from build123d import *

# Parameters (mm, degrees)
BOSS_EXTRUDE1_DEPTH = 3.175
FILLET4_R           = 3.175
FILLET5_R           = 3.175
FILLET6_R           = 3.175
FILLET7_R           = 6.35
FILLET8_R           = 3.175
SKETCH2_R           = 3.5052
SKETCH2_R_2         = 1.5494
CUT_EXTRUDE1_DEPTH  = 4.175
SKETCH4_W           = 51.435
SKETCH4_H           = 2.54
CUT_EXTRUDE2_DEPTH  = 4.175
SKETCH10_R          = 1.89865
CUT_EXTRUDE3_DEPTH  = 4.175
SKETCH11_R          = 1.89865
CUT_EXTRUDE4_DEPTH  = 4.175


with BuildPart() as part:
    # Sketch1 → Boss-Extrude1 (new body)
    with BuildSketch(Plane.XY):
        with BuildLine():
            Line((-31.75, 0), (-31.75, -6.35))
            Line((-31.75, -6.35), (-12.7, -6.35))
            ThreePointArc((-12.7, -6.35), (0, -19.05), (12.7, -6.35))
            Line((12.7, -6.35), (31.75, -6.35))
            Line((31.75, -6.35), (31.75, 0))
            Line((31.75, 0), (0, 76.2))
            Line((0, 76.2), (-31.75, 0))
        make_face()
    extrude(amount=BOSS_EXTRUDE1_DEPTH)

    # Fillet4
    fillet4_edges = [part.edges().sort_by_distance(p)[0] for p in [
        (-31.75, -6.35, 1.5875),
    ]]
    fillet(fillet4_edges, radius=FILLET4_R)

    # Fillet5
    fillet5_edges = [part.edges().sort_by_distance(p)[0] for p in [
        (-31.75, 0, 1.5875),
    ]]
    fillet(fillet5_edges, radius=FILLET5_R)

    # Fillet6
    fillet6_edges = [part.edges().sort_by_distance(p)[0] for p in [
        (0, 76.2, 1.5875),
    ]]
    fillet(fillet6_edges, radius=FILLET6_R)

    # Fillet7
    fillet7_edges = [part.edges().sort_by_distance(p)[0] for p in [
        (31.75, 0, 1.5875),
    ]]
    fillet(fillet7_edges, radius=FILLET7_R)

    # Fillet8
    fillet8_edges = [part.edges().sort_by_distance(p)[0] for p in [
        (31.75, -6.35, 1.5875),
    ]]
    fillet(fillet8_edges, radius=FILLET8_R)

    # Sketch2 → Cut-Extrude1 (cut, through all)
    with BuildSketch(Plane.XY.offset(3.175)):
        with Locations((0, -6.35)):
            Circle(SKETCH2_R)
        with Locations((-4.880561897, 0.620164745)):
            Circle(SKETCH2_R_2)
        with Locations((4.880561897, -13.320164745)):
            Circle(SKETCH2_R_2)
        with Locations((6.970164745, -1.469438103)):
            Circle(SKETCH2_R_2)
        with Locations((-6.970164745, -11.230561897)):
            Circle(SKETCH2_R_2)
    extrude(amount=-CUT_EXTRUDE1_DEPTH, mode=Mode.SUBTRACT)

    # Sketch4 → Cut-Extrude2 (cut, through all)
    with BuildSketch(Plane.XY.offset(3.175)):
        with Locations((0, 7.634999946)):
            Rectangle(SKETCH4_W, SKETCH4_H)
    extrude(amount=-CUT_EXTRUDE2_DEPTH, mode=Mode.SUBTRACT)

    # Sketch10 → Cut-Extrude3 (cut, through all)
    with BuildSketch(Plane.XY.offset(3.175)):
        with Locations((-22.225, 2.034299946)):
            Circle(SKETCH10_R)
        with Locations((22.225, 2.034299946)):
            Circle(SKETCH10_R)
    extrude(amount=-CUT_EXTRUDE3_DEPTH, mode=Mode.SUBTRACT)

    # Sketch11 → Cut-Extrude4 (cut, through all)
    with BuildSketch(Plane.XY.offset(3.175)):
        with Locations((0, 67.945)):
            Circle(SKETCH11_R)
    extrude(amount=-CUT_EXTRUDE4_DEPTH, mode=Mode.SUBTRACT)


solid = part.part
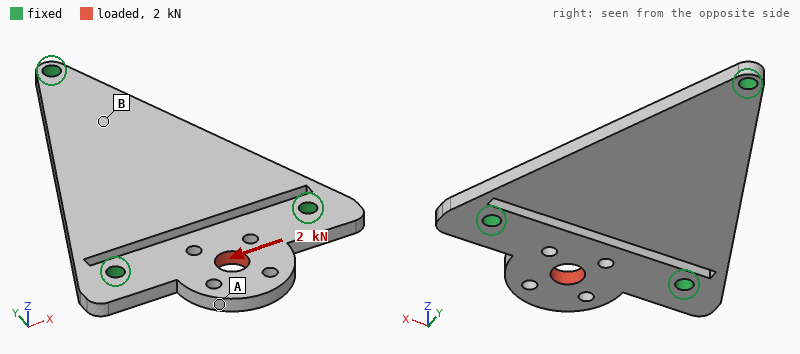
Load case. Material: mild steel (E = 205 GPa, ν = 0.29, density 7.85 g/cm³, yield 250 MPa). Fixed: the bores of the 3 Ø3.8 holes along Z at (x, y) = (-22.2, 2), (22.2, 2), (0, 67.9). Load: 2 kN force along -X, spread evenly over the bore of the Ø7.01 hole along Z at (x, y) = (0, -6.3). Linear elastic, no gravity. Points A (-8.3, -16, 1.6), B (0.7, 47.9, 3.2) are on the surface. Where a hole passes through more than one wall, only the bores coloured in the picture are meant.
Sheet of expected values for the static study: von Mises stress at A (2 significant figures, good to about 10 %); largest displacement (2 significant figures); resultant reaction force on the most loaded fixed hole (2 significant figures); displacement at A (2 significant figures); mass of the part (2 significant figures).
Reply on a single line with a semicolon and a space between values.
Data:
14 MPa; 5.0 µm; 1.1 kN; 4.4 µm; 70 g
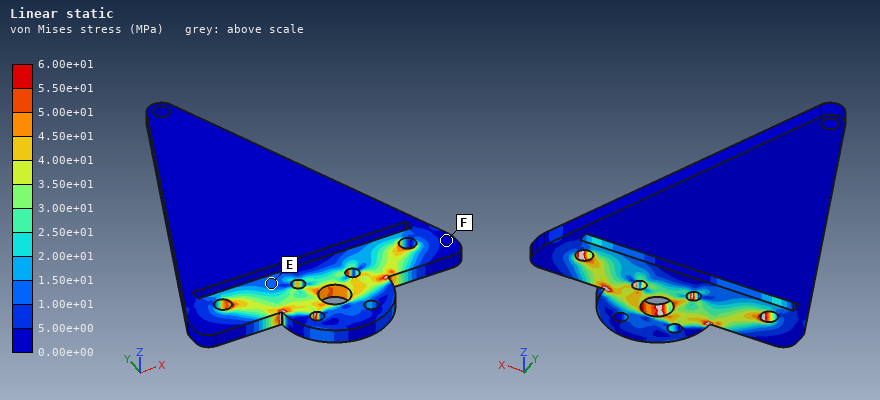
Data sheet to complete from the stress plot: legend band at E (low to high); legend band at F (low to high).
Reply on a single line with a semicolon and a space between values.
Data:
1.00e+01 to 1.50e+01 MPa; 0.00e+00 to 5.00e+00 MPa
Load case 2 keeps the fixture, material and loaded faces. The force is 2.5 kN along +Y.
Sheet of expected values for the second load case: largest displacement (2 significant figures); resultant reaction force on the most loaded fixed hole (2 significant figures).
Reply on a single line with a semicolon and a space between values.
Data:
16 µm; 1.4 kN
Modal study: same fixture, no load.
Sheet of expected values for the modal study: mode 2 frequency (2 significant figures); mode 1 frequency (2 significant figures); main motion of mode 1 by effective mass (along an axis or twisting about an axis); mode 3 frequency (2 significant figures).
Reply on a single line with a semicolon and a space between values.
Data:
4600 Hz; 2400 Hz; along Z; 4700 Hz
